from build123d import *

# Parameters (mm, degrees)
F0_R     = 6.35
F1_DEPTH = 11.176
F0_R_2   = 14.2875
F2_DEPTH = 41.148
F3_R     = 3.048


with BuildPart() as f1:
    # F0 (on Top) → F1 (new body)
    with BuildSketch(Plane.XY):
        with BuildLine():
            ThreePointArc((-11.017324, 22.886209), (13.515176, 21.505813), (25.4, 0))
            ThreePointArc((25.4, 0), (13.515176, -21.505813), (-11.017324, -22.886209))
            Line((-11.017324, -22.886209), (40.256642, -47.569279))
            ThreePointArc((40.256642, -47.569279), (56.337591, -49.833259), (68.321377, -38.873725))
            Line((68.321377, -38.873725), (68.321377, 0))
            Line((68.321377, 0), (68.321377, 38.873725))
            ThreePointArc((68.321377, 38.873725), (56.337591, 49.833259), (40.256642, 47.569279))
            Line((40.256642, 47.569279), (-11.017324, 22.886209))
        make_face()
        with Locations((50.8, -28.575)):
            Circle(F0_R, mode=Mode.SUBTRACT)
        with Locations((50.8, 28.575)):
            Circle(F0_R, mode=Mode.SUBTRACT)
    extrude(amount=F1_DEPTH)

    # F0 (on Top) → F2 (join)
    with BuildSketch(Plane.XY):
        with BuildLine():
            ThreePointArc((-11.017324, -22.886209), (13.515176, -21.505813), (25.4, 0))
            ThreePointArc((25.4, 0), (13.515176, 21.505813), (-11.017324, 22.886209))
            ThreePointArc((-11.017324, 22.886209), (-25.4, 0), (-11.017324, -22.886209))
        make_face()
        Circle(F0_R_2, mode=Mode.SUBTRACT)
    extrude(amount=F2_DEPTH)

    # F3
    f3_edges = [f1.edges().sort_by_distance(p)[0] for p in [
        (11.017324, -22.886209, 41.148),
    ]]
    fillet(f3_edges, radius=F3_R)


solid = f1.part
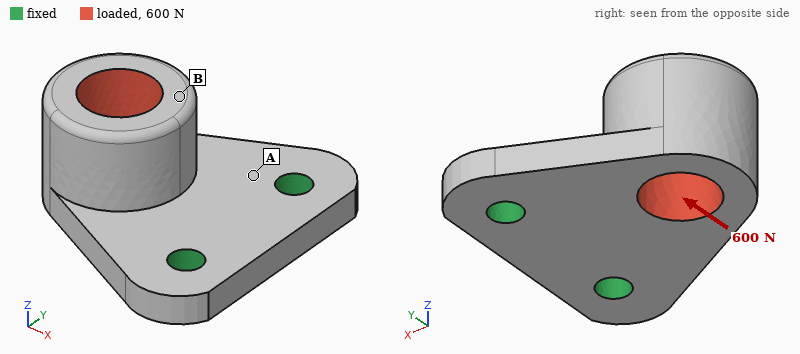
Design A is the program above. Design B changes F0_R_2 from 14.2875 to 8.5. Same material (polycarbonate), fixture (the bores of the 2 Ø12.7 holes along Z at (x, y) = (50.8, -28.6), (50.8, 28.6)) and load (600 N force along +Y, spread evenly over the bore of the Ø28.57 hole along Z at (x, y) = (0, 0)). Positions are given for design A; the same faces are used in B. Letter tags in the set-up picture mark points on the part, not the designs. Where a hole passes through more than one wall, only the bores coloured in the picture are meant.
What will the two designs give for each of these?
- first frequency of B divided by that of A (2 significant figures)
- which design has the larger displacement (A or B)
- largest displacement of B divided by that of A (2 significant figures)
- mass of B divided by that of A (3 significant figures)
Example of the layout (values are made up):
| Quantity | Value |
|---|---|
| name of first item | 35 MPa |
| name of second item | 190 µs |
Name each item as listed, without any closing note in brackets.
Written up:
| Quantity | Value |
|---|---|
| first frequency of B divided by that of A | 0.90 |
| which design has the larger displacement | A |
| largest displacement of B divided by that of A | 0.88 |
| mass of B divided by that of A | 1.16 |
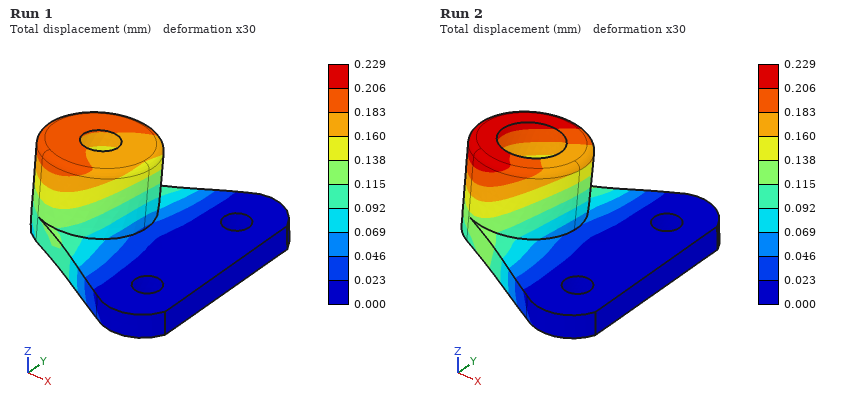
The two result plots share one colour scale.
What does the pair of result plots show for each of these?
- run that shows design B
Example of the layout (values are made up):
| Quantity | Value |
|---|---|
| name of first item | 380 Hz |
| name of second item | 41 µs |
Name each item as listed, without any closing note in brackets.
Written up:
| Quantity | Value |
|---|---|
| run that shows design B | Run 1 |
